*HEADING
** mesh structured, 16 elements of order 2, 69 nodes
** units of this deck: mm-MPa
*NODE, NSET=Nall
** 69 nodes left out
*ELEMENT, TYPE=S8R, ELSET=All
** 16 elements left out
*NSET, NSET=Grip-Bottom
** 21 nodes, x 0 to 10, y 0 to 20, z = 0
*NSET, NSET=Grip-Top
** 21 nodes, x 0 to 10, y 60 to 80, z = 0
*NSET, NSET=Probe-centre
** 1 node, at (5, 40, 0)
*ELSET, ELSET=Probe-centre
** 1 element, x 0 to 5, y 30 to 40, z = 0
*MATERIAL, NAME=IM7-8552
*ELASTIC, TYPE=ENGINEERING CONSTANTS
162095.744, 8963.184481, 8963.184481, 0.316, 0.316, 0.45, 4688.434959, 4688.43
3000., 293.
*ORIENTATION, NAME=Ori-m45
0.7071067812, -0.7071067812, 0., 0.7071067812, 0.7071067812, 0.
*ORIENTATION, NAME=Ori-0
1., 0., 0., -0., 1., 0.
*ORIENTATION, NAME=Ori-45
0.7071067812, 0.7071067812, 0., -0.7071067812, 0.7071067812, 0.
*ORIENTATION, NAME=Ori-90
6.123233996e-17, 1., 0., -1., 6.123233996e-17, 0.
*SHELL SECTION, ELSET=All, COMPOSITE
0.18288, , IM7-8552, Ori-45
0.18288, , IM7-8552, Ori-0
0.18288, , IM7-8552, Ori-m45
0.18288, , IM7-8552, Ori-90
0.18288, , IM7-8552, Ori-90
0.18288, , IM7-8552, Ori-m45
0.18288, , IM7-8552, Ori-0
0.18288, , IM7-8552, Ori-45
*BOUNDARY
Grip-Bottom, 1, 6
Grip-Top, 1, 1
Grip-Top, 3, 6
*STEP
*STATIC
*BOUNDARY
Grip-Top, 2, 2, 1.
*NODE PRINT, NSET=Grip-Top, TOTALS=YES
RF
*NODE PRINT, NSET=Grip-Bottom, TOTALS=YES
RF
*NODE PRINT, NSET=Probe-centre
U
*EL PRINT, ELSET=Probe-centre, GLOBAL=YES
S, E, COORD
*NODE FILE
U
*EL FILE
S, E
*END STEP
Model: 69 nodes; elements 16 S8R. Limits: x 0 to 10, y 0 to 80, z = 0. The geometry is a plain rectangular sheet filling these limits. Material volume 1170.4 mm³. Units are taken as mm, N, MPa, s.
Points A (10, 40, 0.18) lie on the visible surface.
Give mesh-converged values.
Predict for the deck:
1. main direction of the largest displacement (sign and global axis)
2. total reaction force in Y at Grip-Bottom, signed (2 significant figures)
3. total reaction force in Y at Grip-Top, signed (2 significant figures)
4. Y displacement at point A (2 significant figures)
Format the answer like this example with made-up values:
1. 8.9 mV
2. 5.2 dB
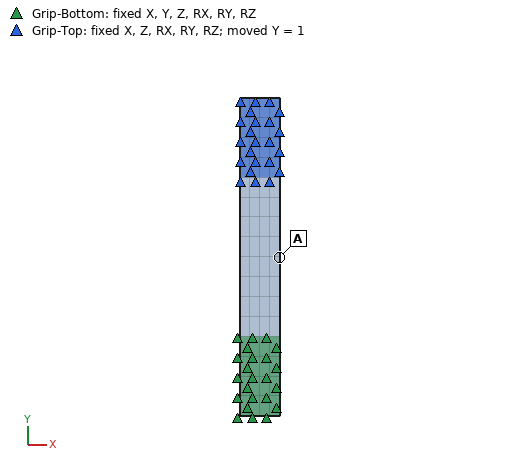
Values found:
1. +Y
2. -22000 N
3. 22000 N
4. 0.51 mm
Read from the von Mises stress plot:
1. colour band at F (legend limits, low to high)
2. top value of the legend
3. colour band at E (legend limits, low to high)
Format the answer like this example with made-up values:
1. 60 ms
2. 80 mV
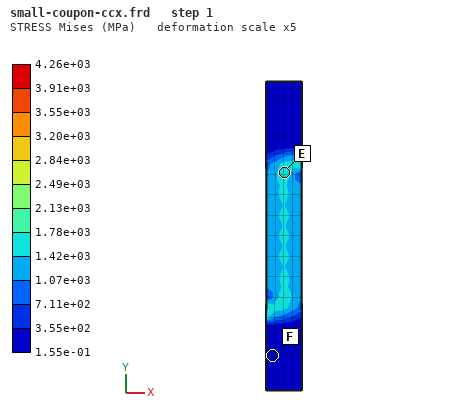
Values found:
1. 1.55e-01 to 3.55e+02 MPa
2. 4.26e+03 MPa
3. 1.42e+03 to 1.78e+03 MPa
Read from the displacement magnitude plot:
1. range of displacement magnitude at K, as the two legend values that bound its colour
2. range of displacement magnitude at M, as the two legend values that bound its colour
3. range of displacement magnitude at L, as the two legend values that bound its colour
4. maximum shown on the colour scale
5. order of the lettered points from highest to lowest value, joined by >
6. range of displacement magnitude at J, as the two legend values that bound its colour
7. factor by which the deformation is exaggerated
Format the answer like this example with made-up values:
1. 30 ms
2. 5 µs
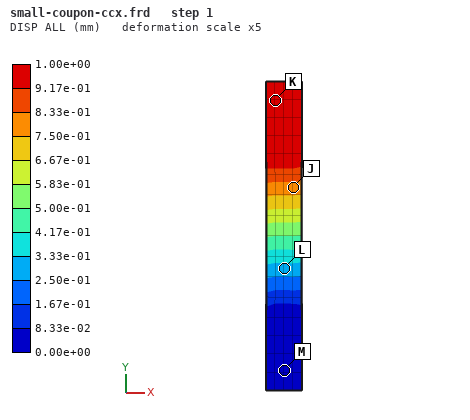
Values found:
1. 9.17e-01 to 1.00e+00 mm
2. 0.00e+00 to 8.33e-02 mm
3. 2.50e-01 to 3.33e-01 mm
4. 1.00e+00 mm
5. K > J > L > M
6. 7.50e-01 to 8.33e-01 mm
7. 5
